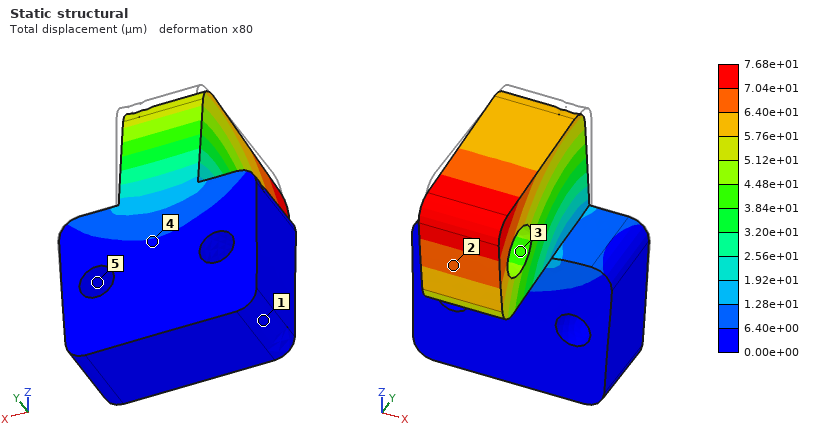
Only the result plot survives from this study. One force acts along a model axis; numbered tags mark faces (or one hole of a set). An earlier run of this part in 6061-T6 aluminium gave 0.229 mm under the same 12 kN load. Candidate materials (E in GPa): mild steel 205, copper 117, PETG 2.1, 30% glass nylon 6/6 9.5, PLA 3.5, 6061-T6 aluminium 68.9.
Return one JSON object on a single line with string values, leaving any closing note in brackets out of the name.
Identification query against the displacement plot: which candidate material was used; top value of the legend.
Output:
{"which candidate material was used": "mild steel", "top value of the legend": "7.68e+01 µm"}
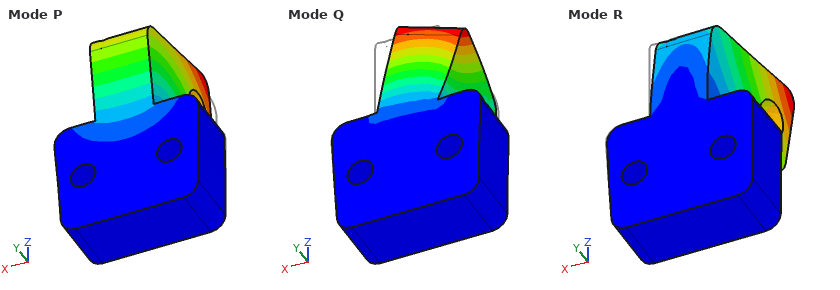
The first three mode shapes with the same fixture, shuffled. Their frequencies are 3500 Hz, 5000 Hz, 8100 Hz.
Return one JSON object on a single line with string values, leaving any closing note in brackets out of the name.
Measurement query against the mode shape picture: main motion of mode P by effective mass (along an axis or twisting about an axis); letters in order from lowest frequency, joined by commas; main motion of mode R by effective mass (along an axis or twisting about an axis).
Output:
{"main motion of mode P by effective mass": "along Y", "letters in order from lowest frequency, joined by commas": "P, R, Q", "main motion of mode R by effective mass": "along X"}
